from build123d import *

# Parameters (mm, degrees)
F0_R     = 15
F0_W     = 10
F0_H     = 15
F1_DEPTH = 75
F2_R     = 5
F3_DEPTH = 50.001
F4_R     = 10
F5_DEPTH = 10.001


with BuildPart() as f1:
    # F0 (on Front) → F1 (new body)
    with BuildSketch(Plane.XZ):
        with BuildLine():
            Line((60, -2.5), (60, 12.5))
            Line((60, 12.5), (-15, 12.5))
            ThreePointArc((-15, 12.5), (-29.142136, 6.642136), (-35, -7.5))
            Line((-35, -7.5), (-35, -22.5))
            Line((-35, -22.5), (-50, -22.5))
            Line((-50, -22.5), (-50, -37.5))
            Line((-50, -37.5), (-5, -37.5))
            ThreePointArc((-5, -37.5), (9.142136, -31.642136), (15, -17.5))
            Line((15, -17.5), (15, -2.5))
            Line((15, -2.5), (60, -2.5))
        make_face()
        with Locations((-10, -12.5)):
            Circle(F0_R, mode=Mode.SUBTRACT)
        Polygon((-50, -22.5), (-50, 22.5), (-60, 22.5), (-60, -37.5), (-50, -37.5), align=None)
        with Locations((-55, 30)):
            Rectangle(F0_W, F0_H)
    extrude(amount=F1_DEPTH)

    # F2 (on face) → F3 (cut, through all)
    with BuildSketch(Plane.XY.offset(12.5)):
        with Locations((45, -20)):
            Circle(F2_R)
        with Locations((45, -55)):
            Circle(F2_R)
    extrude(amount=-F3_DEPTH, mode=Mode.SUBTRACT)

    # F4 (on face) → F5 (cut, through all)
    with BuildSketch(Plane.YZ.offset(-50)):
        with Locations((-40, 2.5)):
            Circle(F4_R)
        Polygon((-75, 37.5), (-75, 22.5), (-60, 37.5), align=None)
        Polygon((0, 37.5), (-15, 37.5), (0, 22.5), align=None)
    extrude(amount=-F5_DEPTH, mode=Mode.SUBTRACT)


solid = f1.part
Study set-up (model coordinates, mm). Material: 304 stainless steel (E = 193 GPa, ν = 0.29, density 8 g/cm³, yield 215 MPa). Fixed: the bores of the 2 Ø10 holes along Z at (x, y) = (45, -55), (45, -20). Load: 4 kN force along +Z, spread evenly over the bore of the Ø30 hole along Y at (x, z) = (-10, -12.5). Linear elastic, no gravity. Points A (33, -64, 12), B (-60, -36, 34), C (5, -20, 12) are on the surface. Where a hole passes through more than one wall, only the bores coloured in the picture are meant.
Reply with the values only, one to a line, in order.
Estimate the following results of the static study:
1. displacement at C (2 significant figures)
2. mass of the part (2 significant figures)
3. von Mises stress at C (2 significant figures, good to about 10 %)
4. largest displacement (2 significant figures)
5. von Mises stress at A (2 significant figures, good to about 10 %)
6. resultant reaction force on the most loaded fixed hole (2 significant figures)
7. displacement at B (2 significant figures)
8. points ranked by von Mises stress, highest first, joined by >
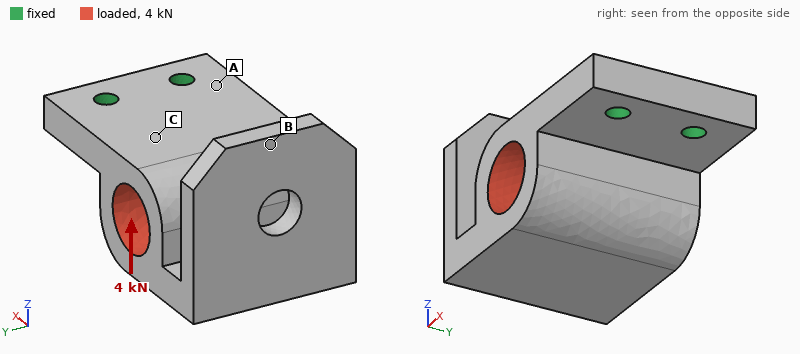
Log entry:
0.034 mm
1.9 kg
16 MPa
0.14 mm
54 MPa
2.0 kN
0.13 mm
A > C > B
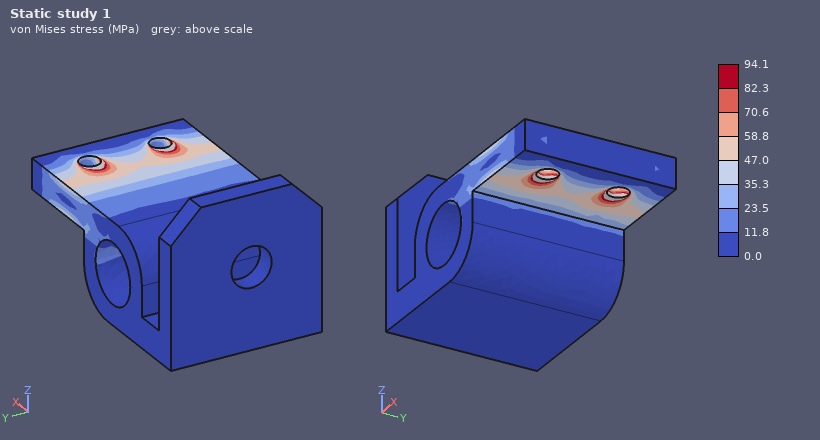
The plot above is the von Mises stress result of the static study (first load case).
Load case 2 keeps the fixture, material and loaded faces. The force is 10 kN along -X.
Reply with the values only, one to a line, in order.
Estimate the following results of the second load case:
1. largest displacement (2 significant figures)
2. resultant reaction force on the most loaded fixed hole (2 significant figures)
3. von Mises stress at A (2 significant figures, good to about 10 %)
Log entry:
0.16 mm
5.0 kN
47 MPa
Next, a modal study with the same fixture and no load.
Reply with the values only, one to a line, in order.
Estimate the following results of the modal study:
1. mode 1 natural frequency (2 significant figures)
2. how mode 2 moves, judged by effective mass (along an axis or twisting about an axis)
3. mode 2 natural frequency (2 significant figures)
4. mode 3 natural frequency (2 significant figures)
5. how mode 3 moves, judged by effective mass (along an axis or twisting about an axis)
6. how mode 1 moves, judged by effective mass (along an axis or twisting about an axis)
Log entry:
660 Hz
along X
1600 Hz
1900 Hz
along Y
along Z
